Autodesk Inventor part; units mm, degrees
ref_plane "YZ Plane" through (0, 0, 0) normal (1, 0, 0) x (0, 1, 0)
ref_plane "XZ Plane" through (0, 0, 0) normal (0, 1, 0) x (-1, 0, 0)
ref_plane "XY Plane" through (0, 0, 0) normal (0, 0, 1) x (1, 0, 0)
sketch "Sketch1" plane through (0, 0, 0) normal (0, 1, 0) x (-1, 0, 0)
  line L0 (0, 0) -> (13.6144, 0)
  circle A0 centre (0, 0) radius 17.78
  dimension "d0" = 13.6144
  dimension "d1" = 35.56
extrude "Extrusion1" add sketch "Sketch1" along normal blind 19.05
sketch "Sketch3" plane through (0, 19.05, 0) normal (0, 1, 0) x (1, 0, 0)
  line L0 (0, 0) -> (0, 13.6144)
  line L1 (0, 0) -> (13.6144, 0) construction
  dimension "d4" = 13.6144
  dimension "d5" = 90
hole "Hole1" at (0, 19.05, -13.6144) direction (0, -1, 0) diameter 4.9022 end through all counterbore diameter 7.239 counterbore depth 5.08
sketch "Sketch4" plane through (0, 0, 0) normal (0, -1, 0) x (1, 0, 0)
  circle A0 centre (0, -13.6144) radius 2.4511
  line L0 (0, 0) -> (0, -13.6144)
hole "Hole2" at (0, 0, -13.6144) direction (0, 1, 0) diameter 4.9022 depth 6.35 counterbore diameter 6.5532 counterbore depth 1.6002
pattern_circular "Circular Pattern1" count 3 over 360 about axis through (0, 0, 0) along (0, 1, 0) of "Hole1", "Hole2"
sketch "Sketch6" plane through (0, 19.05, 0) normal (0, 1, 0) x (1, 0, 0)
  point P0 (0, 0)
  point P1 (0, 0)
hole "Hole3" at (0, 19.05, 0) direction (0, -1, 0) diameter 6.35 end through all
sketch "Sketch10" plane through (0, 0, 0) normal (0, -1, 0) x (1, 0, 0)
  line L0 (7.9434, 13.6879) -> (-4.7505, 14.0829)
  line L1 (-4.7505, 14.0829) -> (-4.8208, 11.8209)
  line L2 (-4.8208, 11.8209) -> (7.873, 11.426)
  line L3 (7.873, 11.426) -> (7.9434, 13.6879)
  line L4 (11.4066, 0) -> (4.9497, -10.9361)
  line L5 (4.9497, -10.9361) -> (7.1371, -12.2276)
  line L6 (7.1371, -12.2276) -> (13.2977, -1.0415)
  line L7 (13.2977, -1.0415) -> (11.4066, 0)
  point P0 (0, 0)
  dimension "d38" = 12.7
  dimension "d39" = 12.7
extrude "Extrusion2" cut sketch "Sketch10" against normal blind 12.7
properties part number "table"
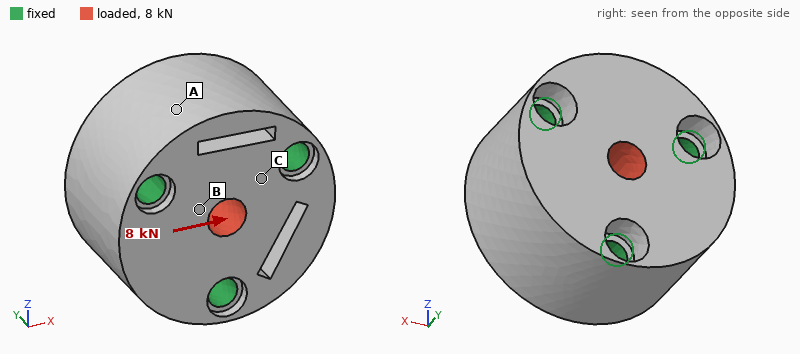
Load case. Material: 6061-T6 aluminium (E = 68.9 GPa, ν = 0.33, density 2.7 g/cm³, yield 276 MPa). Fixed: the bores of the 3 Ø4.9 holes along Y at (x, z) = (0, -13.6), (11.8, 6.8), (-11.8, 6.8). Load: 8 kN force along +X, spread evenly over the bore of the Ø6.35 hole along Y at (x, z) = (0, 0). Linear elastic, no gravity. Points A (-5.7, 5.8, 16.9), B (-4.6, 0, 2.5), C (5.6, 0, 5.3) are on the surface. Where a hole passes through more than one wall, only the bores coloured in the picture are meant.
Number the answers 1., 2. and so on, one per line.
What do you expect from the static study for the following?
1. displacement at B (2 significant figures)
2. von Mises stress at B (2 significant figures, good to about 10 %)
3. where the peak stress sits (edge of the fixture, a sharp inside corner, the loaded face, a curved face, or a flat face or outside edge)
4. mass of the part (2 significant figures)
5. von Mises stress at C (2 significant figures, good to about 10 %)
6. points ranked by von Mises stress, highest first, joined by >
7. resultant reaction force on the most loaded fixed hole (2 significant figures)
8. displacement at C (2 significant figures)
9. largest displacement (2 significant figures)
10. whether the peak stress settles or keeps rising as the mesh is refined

1. 2.3 µm
2. 20 MPa
3. edge of the fixture
4. 43 g
5. 12 MPa
6. B > C > A
7. 2.9 kN
8. 1.4 µm
9. 5.0 µm
10. keeps rising
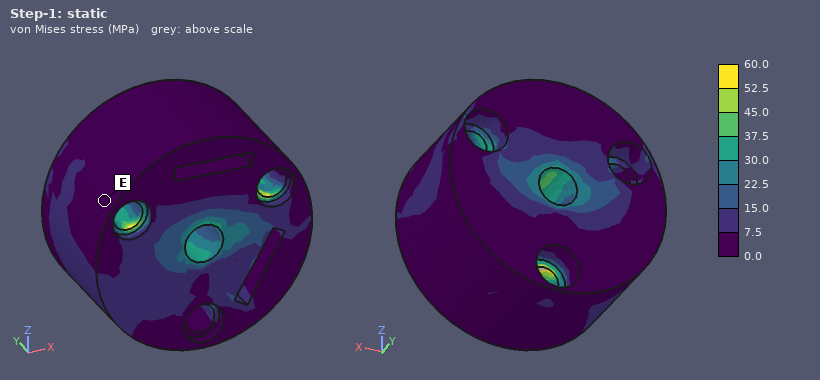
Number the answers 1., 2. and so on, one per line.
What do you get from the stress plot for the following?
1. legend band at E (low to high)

1. 0.0 to 7.5 MPa
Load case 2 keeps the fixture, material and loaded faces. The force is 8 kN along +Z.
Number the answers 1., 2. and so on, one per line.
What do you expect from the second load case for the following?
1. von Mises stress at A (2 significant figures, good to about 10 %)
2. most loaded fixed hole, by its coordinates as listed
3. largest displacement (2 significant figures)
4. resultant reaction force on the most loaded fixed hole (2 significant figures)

1. 10.0 MPa
2. (0, -13.6)
3. 5.4 µm
4. 3.1 kN
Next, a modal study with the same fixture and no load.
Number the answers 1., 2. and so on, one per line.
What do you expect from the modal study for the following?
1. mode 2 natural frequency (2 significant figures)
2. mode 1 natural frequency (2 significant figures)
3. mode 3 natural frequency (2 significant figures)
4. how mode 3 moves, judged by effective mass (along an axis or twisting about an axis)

1. 39 kHz
2. 38 kHz
3. 45 kHz
4. along Y
